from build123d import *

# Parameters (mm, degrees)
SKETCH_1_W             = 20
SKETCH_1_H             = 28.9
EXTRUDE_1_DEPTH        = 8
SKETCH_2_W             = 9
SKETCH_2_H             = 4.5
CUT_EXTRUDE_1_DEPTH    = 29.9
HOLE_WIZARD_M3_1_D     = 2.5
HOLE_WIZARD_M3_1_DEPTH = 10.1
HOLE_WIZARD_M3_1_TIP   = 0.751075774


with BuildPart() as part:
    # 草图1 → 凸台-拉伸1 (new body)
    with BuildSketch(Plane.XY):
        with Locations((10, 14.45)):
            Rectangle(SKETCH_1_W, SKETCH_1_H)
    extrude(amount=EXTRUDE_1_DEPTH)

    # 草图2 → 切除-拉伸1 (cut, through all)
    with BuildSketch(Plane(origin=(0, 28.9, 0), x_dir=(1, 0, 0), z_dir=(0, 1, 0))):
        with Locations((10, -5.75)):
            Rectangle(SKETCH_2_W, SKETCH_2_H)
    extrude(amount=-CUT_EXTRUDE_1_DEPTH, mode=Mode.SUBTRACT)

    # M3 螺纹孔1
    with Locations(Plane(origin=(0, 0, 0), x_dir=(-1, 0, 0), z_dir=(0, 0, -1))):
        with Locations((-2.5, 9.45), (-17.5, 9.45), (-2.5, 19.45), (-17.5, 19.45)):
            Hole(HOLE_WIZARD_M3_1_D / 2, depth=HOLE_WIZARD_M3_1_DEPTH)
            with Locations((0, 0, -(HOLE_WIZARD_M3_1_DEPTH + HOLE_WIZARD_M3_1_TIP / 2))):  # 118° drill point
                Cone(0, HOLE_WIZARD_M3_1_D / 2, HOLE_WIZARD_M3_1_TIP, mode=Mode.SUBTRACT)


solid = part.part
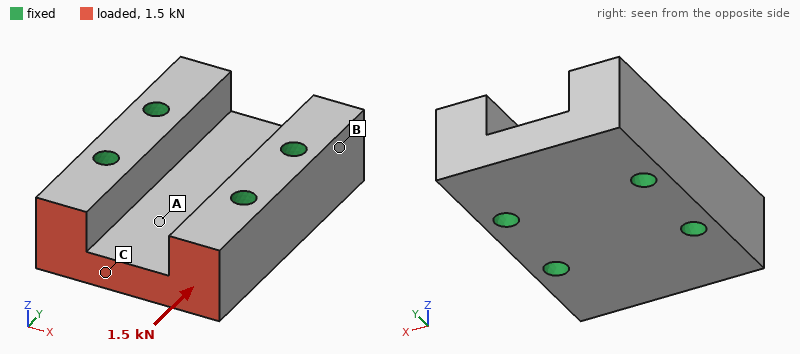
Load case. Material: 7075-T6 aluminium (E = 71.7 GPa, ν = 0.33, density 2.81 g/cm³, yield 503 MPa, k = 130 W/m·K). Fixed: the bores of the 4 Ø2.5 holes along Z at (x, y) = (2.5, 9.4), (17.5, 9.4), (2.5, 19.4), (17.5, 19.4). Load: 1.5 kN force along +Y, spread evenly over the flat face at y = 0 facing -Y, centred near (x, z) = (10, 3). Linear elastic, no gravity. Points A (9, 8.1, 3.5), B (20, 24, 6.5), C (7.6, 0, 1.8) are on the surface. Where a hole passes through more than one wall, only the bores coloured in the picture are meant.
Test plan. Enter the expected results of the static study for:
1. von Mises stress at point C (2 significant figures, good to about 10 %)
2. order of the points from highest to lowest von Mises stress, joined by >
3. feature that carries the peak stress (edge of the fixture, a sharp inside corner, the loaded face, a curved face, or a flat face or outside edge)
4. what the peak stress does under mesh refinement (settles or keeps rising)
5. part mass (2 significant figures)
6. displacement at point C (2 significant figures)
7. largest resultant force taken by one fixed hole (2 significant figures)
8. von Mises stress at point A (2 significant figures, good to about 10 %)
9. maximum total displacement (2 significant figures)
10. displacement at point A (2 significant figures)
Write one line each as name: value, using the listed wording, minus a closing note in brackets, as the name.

von Mises stress at point C: 11 MPa
order of the points from highest to lowest von Mises stress, joined by >: C > A > B
feature that carries the peak stress: edge of the fixture
what the peak stress does under mesh refinement: keeps rising
part mass: 9.3 g
displacement at point C: 2.0 µm
largest resultant force taken by one fixed hole: 670 N
von Mises stress at point A: 6.4 MPa
maximum total displacement: 2.2 µm
displacement at point A: 0.84 µm
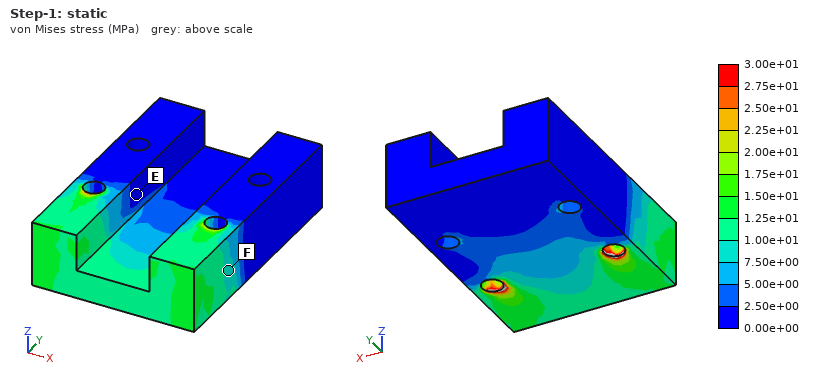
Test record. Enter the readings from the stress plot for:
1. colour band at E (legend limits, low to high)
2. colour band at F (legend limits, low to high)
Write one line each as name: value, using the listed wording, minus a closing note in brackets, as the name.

colour band at E: 0.00e+00 to 2.50e+00 MPa
colour band at F: 7.50e+00 to 1.00e+01 MPa
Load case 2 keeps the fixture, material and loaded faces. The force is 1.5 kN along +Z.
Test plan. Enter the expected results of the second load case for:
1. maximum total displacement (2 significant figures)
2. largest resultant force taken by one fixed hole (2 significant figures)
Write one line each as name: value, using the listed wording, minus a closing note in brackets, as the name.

maximum total displacement: 22 µm
largest resultant force taken by one fixed hole: 820 N
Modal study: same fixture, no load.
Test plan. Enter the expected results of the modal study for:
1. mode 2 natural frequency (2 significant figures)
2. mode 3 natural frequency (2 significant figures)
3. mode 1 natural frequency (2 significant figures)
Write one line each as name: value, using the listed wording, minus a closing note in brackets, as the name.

mode 2 natural frequency: 48 kHz
mode 3 natural frequency: 55 kHz
mode 1 natural frequency: 47 kHz
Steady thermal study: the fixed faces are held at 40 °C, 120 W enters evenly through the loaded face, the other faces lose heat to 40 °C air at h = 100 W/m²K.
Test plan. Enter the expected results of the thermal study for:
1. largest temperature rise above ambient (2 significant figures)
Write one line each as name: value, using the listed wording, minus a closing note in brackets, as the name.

largest temperature rise above ambient: 74 K
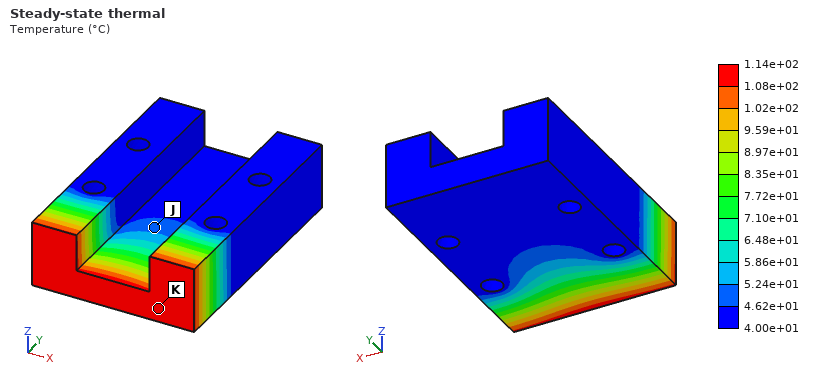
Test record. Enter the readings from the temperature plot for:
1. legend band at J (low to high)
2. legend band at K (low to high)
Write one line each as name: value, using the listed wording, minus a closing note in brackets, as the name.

legend band at J: 4.62e+01 to 5.24e+01 °C
legend band at K: 1.08e+02 to 1.14e+02 °C
